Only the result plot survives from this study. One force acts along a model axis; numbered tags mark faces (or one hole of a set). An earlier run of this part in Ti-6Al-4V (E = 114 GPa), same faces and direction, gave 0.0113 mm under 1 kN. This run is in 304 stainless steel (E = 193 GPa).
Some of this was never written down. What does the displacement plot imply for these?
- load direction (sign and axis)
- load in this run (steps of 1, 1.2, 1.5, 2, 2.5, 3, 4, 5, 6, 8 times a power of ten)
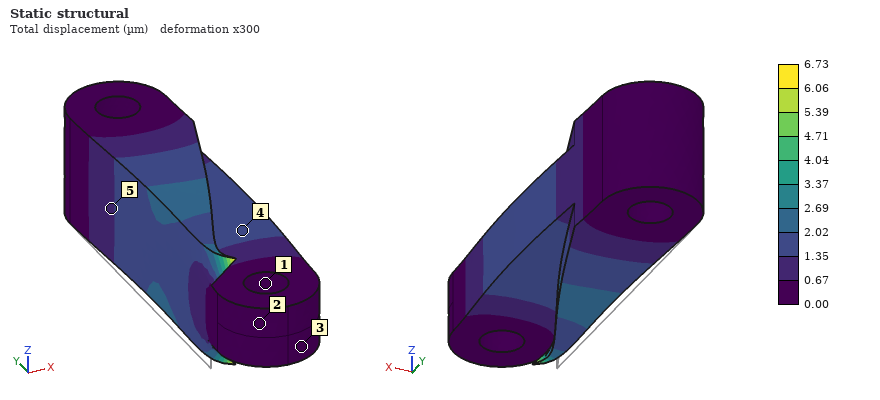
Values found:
+X
1 kN
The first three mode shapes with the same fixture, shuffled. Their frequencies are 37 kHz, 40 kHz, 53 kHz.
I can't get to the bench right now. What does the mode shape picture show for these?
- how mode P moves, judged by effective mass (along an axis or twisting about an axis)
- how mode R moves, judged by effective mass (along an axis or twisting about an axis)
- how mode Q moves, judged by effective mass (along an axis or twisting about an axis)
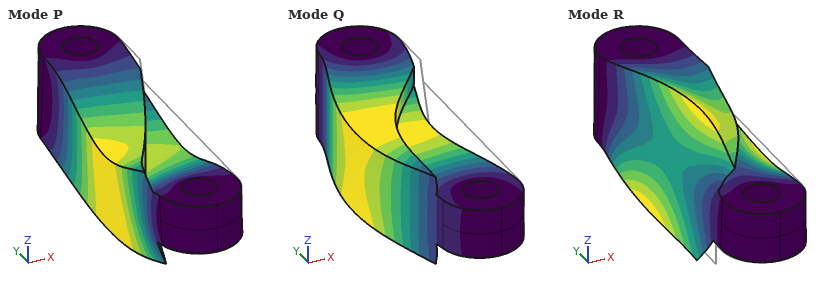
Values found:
along Z
twisting about Y
along X
